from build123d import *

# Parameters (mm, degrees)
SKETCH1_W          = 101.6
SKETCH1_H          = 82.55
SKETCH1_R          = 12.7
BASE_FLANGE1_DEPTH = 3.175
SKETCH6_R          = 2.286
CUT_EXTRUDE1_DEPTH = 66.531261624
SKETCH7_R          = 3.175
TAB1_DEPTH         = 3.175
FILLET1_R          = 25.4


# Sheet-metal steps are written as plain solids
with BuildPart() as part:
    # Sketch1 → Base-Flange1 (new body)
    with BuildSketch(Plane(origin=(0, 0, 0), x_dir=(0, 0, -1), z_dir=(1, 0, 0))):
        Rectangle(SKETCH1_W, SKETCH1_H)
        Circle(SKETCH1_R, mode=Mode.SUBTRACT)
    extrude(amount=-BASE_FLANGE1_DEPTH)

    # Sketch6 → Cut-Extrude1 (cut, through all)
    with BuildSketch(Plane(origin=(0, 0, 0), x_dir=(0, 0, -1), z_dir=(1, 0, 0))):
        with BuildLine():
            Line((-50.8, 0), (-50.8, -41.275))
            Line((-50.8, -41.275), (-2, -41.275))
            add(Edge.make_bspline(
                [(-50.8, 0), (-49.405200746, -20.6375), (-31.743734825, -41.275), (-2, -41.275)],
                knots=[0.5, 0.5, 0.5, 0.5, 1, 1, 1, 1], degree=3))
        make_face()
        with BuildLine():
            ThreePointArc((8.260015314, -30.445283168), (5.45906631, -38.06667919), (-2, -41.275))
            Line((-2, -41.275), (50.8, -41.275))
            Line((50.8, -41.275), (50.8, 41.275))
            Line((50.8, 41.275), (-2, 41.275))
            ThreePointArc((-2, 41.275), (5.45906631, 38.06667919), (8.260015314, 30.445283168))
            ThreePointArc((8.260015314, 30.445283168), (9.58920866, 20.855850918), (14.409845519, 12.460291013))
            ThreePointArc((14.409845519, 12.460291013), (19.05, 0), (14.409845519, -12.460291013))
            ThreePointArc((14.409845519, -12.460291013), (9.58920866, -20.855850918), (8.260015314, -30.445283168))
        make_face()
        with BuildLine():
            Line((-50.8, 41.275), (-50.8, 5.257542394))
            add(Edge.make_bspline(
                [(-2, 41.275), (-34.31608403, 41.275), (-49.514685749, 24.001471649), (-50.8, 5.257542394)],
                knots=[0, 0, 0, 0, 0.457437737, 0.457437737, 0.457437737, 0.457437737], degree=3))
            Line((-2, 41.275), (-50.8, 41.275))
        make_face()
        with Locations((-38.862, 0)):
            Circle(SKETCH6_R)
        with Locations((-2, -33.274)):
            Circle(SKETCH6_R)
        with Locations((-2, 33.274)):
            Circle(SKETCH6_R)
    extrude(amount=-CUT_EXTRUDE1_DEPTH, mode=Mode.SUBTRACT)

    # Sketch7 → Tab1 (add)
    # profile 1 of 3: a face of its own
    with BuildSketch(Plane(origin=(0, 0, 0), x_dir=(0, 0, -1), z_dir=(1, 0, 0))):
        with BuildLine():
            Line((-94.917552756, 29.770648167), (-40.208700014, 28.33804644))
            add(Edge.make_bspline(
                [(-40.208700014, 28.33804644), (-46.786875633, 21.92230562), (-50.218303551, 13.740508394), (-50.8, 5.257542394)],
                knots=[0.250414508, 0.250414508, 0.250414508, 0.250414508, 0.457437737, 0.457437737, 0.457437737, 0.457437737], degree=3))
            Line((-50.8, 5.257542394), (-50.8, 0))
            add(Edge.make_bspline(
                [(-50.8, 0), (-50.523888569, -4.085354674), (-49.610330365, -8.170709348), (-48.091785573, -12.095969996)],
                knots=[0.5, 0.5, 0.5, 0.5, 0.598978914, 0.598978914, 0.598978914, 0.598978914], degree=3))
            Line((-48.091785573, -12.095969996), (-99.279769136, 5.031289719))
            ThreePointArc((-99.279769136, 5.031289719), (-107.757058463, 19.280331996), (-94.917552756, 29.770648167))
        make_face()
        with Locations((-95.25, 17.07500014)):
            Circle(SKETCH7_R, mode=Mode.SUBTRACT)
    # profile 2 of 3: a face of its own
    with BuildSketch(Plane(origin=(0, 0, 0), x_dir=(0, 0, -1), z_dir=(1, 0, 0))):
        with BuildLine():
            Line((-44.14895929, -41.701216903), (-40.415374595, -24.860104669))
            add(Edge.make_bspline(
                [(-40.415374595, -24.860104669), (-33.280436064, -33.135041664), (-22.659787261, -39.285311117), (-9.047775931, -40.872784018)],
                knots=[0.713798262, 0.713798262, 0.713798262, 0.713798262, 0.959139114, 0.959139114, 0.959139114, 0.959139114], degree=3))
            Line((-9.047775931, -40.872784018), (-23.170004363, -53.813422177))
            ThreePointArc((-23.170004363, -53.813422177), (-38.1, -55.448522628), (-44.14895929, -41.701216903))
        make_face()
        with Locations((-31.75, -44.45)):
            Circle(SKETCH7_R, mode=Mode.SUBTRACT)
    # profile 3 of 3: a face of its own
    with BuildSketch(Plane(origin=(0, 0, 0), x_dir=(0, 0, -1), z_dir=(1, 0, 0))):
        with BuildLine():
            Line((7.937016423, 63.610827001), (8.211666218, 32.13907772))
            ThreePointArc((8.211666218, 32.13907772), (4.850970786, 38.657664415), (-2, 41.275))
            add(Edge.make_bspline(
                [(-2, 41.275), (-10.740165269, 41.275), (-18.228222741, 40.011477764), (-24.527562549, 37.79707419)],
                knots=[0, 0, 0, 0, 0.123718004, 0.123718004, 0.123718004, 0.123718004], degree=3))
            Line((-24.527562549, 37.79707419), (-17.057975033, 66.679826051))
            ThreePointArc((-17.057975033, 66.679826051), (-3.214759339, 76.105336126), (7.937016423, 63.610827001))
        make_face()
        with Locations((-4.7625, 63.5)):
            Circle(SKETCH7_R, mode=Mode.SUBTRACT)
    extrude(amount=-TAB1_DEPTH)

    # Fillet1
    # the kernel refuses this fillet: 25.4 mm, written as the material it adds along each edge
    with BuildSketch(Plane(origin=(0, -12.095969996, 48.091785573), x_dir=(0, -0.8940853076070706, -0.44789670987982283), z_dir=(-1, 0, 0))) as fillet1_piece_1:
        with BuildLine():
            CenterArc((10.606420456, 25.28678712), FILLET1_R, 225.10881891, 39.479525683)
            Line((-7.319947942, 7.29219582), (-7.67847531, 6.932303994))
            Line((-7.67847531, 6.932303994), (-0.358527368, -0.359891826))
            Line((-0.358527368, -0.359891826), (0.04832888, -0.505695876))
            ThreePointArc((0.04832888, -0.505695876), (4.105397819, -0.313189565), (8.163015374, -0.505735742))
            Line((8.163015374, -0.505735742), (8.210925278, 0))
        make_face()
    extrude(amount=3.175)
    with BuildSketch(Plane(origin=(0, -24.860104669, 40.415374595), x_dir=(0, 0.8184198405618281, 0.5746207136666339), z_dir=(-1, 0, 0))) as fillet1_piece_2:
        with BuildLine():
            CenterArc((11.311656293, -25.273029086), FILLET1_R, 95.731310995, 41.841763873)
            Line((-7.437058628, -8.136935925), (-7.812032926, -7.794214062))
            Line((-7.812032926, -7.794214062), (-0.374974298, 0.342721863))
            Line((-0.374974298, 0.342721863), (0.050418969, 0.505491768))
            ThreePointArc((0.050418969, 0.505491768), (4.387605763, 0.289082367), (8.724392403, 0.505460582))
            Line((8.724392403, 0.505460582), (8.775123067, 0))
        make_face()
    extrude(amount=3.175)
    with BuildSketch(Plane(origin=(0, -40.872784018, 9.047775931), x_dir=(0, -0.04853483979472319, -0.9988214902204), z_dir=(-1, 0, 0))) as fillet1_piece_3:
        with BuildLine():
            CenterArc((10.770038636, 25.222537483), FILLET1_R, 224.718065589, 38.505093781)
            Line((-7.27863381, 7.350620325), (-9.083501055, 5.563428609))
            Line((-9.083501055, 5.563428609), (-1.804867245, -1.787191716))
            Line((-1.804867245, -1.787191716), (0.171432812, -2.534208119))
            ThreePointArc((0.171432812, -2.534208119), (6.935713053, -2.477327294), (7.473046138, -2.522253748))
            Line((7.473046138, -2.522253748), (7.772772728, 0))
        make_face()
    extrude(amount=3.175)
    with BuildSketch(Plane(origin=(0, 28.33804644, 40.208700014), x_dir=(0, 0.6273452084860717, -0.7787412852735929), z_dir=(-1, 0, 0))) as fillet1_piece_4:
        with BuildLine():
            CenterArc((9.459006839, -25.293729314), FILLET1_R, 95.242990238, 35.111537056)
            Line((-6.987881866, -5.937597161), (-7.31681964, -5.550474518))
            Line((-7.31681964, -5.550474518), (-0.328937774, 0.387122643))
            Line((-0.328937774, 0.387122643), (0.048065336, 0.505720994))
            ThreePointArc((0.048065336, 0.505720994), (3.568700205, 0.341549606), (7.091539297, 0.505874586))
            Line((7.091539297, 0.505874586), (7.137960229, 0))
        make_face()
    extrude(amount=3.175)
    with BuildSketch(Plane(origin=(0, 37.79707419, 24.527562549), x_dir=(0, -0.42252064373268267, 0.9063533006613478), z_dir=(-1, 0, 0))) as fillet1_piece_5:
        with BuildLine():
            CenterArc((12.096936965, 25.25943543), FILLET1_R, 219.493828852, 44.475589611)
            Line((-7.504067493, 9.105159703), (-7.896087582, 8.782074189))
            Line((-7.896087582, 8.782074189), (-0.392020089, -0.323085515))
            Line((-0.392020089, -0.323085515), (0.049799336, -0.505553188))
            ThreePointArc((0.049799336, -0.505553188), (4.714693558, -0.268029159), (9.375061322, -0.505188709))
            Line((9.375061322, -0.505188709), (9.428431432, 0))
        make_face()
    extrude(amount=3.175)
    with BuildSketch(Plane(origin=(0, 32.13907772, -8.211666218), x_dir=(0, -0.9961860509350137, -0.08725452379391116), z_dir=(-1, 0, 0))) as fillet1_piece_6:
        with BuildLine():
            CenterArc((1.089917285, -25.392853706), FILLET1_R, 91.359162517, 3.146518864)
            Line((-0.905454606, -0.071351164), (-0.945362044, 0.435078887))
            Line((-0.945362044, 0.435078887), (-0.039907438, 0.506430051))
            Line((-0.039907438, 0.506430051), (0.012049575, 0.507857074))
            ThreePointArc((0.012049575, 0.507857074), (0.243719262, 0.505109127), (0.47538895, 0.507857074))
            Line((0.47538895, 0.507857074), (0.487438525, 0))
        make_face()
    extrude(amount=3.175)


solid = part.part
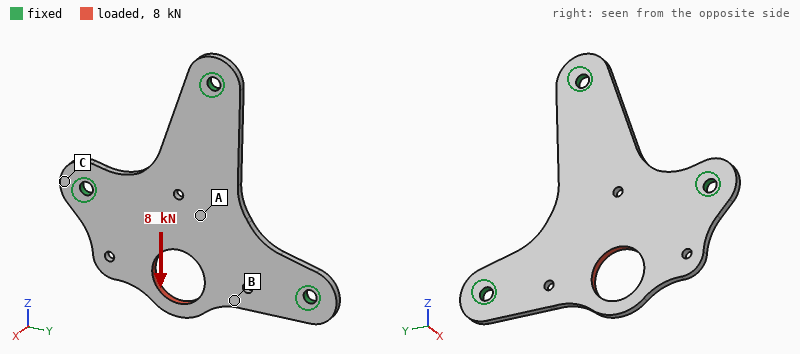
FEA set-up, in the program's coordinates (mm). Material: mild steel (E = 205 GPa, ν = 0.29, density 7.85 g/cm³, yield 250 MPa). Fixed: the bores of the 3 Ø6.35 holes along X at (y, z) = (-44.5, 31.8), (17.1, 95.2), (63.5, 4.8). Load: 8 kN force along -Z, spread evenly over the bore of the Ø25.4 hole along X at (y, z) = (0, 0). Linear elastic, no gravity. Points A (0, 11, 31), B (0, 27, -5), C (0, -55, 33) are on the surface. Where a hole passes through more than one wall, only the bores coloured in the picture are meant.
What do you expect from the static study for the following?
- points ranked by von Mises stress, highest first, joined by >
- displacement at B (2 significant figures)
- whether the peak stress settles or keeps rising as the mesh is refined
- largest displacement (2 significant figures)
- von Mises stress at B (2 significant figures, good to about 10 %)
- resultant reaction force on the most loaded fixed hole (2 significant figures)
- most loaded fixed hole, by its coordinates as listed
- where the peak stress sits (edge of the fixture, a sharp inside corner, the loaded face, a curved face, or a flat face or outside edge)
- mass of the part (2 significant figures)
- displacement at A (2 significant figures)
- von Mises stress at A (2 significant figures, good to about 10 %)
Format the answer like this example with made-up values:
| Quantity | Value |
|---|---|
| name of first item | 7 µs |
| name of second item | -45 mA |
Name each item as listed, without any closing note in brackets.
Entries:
| Quantity | Value |
|---|---|
| points ranked by von Mises stress, highest first, joined by > | A > B > C |
| displacement at B | 17 µm |
| whether the peak stress settles or keeps rising as the mesh is refined | keeps rising |
| largest displacement | 29 µm |
| von Mises stress at B | 31 MPa |
| resultant reaction force on the most loaded fixed hole | 4.3 kN |
| most loaded fixed hole, by its coordinates as listed | (17.1, 95.2) |
| where the peak stress sits | edge of the fixture |
| mass of the part | 180 g |
| displacement at A | 15 µm |
| von Mises stress at A | 53 MPa |
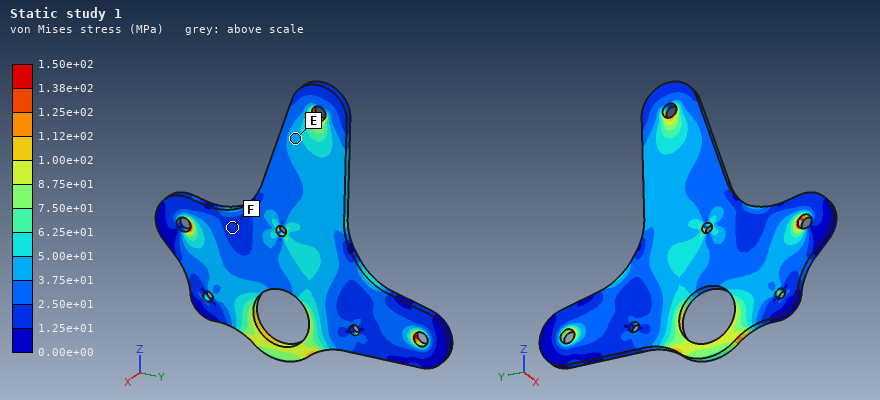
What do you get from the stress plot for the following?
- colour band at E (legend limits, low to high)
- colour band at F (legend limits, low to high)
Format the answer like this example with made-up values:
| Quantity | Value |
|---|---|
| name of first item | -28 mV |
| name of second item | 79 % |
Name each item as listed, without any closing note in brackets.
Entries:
| Quantity | Value |
|---|---|
| colour band at E | 3.75e+01 to 5.00e+01 MPa |
| colour band at F | 1.25e+01 to 2.50e+01 MPa |
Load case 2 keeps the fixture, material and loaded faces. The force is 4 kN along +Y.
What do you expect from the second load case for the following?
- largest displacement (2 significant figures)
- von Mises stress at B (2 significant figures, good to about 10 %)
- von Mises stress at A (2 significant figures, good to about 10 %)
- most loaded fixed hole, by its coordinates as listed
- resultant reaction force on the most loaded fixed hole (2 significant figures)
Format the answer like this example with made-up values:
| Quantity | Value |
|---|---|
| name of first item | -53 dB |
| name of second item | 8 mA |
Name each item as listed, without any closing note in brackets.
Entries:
| Quantity | Value |
|---|---|
| largest displacement | 16 µm |
| von Mises stress at B | 45 MPa |
| von Mises stress at A | 9.1 MPa |
| most loaded fixed hole, by its coordinates as listed | (-44.5, 31.8) |
| resultant reaction force on the most loaded fixed hole | 2.2 kN |
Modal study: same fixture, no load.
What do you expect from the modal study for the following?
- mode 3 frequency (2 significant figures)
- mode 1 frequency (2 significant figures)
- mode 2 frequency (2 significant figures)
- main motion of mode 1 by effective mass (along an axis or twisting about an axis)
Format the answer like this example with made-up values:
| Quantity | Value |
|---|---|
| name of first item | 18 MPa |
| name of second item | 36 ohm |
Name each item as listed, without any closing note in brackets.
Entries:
| Quantity | Value |
|---|---|
| mode 3 frequency | 2900 Hz |
| mode 1 frequency | 1200 Hz |
| mode 2 frequency | 1700 Hz |
| main motion of mode 1 by effective mass | along X |
